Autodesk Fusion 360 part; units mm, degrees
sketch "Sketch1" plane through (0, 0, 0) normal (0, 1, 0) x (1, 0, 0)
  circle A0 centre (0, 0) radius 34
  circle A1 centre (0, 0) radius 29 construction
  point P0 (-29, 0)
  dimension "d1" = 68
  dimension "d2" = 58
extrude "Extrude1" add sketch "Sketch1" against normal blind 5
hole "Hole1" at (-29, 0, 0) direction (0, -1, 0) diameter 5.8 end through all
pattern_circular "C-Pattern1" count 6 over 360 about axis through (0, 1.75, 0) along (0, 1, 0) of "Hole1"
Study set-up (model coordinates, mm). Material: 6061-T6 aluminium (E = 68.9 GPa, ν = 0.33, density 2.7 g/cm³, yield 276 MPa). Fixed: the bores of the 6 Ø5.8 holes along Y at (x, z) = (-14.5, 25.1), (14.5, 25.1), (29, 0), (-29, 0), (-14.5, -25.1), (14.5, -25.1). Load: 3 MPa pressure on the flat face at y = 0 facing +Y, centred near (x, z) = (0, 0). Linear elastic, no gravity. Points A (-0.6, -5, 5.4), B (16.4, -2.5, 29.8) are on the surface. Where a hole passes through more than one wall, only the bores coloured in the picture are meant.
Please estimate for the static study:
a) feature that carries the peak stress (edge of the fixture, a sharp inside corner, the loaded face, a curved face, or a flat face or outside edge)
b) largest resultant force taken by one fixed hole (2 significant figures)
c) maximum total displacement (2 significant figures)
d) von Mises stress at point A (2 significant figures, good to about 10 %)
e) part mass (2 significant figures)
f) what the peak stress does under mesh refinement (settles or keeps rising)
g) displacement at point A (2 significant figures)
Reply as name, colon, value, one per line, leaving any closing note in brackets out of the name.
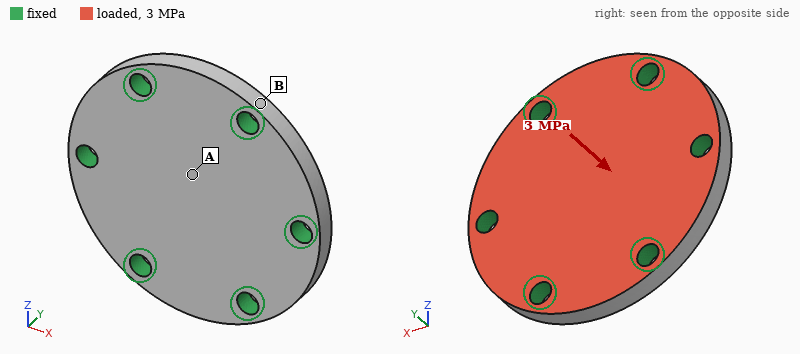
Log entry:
feature that carries the peak stress: edge of the fixture
largest resultant force taken by one fixed hole: 1.7 kN
maximum total displacement: 48 µm
von Mises stress at point A: 46 MPa
part mass: 47 g
what the peak stress does under mesh refinement: keeps rising
displacement at point A: 46 µm
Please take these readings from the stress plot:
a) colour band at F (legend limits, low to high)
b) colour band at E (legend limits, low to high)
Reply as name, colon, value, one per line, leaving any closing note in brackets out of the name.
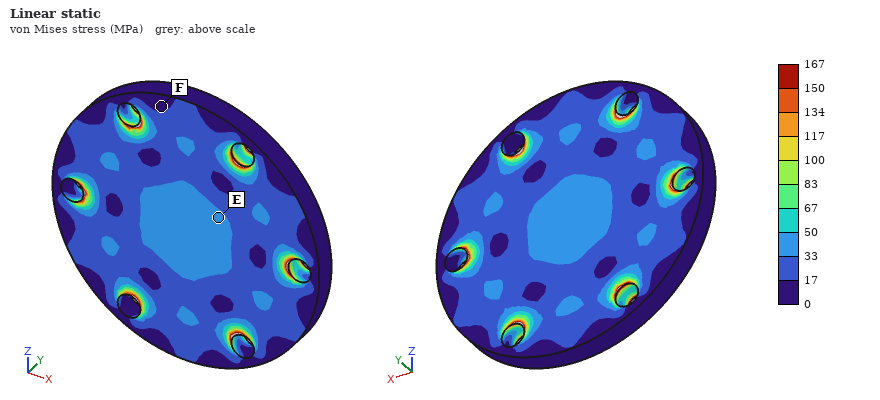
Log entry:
colour band at F: 0 to 17 MPa
colour band at E: 33 to 50 MPa
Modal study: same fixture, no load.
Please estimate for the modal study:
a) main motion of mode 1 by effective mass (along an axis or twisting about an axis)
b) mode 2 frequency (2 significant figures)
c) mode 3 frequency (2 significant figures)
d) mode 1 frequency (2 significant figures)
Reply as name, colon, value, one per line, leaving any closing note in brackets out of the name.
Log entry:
main motion of mode 1 by effective mass: along Y
mode 2 frequency: 25 kHz
mode 3 frequency: 25 kHz
mode 1 frequency: 13 kHz
